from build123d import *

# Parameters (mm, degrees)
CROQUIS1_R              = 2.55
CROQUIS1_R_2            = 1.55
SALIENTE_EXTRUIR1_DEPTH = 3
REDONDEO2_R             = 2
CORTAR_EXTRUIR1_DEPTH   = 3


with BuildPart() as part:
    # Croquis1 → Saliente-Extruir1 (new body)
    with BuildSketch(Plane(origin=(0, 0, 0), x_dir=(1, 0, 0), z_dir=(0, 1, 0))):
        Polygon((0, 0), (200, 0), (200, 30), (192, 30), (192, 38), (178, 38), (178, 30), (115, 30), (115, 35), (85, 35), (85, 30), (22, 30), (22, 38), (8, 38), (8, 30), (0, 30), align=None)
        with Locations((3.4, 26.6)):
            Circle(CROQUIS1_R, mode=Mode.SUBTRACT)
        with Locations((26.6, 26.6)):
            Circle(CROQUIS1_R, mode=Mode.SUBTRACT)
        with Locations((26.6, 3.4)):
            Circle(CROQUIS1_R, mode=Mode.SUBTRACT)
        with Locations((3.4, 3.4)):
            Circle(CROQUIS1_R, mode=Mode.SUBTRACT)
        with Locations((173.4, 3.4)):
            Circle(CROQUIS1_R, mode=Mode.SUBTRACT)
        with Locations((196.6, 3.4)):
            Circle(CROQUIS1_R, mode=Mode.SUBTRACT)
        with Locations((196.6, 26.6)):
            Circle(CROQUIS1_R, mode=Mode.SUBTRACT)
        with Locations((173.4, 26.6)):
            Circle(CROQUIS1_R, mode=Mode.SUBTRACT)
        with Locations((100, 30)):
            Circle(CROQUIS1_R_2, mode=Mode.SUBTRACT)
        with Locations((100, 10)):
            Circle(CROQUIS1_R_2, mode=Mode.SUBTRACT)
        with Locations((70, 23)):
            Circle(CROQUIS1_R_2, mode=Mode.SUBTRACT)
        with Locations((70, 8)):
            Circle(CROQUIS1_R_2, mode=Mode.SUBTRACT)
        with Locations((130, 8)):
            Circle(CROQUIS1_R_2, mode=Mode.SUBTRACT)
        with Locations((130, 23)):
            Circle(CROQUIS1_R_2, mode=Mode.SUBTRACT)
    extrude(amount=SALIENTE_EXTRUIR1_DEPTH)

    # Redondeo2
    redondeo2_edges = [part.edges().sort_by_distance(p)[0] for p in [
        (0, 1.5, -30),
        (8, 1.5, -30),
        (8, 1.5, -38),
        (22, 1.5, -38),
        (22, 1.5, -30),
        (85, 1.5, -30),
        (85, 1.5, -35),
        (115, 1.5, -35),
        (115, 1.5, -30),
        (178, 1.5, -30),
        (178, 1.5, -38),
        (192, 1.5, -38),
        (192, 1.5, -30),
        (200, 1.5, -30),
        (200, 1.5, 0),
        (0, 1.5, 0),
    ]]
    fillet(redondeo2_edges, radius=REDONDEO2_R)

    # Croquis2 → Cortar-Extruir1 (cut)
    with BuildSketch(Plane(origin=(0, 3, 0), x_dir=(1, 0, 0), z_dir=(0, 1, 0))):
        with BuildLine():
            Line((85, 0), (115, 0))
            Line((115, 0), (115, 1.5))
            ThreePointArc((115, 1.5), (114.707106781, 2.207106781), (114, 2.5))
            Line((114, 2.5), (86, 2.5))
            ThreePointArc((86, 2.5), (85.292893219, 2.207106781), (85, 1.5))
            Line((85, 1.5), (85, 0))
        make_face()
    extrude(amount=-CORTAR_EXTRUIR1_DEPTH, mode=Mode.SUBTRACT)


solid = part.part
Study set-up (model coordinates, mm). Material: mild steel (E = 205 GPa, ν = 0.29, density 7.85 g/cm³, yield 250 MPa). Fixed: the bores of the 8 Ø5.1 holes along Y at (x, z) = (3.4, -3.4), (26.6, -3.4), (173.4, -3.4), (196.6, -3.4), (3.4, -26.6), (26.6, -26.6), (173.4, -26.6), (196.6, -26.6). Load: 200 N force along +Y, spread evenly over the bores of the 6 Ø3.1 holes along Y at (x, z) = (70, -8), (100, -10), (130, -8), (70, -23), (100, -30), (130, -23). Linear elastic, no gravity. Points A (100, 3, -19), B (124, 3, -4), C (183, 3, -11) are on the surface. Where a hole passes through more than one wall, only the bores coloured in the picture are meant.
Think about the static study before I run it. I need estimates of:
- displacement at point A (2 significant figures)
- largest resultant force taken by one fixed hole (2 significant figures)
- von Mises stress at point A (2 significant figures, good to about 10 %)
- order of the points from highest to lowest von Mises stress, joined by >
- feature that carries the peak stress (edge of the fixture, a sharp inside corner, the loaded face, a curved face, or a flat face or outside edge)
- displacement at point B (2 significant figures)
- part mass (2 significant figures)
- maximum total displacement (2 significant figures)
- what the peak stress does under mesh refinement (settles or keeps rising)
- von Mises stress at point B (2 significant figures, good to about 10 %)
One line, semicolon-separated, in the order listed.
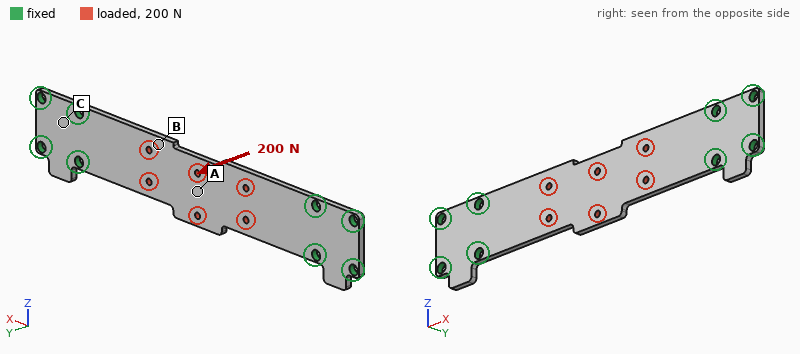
0.17 mm; 68 N; 43 MPa; A > B > C; edge of the fixture; 0.13 mm; 140 g; 0.18 mm; keeps rising; 25 MPa
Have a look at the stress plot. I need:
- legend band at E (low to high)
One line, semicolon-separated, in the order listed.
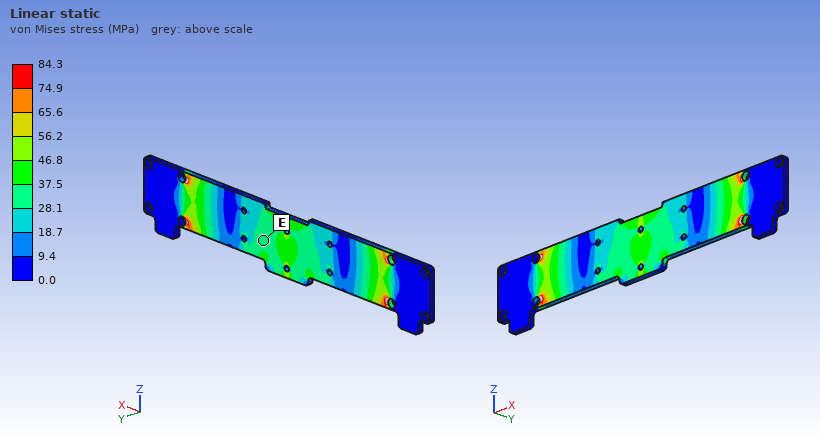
28.1 to 37.5 MPa
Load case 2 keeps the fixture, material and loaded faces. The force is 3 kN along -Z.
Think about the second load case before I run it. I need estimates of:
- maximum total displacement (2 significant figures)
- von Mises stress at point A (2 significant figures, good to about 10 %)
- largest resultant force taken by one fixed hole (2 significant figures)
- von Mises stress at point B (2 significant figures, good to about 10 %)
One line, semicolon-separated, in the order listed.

38 µm; 12 MPa; 2.2 kN; 25 MPa
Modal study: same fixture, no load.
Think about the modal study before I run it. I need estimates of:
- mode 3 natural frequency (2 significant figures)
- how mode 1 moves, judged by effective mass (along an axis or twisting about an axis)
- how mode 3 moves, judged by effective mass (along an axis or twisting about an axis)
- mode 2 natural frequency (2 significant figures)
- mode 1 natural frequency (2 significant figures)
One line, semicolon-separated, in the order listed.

2200 Hz; along Y; twisting about X; 2100 Hz; 740 Hz
